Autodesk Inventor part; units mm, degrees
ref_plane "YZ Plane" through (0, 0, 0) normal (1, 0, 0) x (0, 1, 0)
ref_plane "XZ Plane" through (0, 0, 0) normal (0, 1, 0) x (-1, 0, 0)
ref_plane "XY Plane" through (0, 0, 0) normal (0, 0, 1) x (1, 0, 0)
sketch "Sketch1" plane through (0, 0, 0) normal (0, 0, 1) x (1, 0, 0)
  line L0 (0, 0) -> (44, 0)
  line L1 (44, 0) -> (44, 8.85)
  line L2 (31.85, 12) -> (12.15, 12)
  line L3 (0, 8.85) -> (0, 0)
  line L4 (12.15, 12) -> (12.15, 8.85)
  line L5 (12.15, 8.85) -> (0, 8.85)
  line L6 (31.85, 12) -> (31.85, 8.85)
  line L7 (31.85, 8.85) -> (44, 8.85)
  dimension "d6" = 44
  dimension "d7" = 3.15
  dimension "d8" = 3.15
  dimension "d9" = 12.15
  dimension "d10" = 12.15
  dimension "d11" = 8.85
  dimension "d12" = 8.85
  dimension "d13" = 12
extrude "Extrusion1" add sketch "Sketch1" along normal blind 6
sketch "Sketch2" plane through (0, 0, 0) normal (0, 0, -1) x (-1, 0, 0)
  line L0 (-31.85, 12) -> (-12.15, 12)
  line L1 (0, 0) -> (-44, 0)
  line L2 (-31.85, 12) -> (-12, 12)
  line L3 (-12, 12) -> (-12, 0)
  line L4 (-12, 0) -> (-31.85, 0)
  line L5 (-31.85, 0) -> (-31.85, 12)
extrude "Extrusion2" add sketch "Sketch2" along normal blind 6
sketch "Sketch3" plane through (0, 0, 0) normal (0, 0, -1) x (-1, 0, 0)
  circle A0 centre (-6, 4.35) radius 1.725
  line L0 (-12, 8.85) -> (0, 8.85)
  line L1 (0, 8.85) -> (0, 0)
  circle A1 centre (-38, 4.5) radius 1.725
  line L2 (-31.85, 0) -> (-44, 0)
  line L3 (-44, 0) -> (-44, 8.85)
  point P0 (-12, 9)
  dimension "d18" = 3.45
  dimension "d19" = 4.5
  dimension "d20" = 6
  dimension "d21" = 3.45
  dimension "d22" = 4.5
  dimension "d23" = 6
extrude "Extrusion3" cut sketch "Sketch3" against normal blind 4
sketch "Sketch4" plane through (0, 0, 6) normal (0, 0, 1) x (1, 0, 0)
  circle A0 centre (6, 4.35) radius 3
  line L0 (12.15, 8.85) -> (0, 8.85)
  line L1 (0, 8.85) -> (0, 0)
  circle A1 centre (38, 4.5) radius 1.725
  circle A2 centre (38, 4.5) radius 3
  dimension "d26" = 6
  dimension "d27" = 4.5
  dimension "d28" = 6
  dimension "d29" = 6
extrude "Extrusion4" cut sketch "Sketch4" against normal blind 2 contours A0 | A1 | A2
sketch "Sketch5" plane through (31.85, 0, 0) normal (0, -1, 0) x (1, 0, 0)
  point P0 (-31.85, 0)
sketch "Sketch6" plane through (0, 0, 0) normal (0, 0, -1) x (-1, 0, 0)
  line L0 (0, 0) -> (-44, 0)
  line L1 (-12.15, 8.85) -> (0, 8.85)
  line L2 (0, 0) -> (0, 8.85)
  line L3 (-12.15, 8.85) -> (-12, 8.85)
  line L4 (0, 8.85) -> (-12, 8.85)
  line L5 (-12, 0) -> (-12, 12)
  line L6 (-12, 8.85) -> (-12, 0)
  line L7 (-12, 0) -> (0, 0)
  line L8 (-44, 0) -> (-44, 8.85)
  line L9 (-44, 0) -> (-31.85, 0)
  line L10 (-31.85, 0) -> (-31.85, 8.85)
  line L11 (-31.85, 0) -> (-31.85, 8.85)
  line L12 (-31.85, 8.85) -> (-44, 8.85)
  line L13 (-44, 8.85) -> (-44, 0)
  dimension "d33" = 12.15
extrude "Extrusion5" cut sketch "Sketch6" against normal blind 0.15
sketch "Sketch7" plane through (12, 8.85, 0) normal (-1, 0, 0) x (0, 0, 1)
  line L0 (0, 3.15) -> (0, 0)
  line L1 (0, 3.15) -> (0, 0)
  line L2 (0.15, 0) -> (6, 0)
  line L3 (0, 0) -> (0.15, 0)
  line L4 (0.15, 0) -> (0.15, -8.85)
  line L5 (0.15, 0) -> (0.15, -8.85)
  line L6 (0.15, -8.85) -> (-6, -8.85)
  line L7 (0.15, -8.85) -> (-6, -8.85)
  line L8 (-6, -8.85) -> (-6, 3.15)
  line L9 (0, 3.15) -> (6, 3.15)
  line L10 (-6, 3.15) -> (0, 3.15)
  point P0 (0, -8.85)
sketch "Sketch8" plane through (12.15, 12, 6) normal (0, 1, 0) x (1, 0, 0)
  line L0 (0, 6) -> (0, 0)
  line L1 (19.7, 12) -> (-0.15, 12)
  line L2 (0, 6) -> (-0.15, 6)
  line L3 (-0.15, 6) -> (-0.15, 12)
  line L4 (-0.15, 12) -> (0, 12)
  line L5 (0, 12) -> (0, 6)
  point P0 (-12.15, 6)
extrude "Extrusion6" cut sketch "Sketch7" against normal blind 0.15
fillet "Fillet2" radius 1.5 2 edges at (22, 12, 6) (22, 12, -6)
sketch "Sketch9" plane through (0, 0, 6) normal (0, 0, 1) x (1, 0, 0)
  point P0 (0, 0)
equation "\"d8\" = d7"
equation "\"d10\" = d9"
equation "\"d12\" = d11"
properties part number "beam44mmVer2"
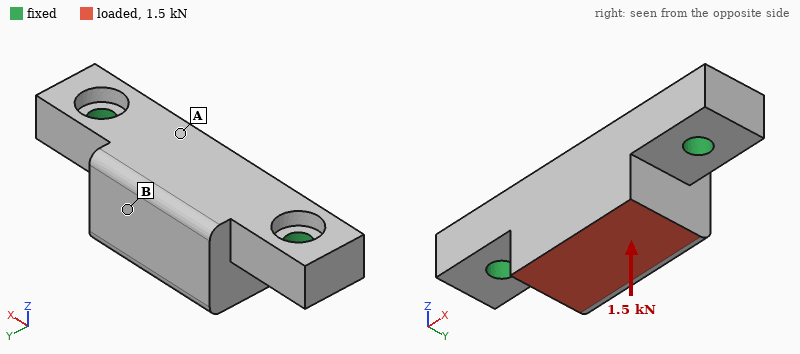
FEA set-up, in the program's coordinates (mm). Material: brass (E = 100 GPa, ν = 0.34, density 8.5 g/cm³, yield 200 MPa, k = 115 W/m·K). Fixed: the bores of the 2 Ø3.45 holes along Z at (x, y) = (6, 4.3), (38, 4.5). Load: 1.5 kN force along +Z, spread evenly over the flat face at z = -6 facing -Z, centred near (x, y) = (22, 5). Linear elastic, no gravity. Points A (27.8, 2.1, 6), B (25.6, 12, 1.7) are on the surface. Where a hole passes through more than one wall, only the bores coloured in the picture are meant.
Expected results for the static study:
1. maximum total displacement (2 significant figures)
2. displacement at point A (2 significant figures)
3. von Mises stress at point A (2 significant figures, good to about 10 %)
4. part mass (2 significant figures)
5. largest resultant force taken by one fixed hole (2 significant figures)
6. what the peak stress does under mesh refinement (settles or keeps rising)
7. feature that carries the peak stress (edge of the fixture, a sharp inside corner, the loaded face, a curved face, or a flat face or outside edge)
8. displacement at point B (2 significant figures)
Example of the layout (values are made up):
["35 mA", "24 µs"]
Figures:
["12 µm", "7.1 µm", "27 MPa", "33 g", "750 N", "keeps rising", "edge of the fixture", "12 µm"]
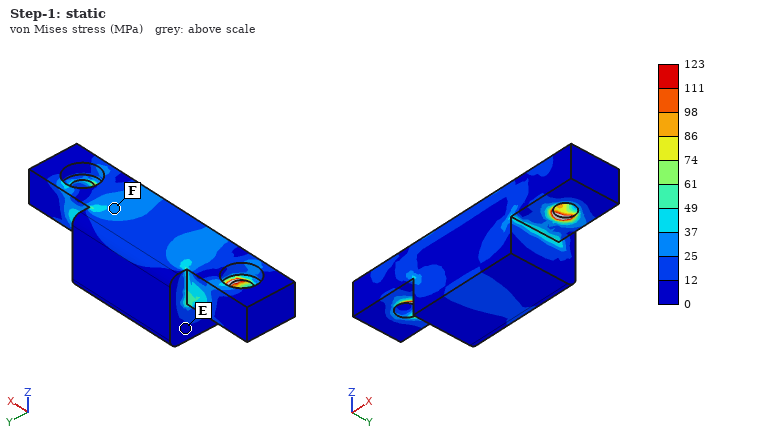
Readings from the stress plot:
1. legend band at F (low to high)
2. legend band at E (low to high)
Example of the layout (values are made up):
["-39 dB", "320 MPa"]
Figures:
["25 to 37 MPa", "0 to 12 MPa"]
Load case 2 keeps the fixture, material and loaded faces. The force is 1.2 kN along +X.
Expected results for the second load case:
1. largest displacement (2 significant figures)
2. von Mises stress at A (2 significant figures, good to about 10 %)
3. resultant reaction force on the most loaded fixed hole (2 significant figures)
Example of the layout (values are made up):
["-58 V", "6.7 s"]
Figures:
["6.2 µm", "8.2 MPa", "710 N"]
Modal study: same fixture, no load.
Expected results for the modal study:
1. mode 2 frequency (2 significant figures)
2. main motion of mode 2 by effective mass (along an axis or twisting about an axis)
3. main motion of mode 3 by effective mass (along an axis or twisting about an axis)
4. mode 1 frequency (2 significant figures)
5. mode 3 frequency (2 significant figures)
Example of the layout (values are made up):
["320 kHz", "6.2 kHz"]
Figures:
["14 kHz", "along Z", "along Y", "8700 Hz", "18 kHz"]
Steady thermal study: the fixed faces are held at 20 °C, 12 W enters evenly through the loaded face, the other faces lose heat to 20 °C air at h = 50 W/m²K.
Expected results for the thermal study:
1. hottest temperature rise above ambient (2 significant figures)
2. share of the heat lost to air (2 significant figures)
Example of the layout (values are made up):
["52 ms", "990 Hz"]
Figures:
["12 K", "4.2 %"]
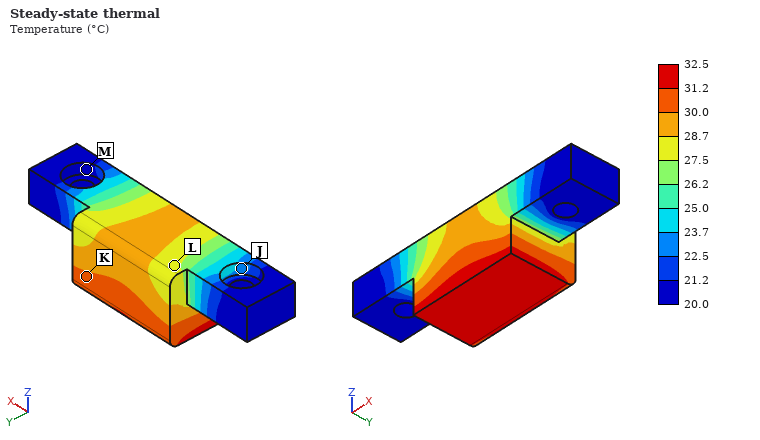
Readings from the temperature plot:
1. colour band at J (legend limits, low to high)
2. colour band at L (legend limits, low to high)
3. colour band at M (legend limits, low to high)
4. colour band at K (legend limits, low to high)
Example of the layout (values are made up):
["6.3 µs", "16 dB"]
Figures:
["22.5 to 23.7 °C", "27.5 to 28.7 °C", "20.0 to 21.2 °C", "30.0 to 31.2 °C"]
